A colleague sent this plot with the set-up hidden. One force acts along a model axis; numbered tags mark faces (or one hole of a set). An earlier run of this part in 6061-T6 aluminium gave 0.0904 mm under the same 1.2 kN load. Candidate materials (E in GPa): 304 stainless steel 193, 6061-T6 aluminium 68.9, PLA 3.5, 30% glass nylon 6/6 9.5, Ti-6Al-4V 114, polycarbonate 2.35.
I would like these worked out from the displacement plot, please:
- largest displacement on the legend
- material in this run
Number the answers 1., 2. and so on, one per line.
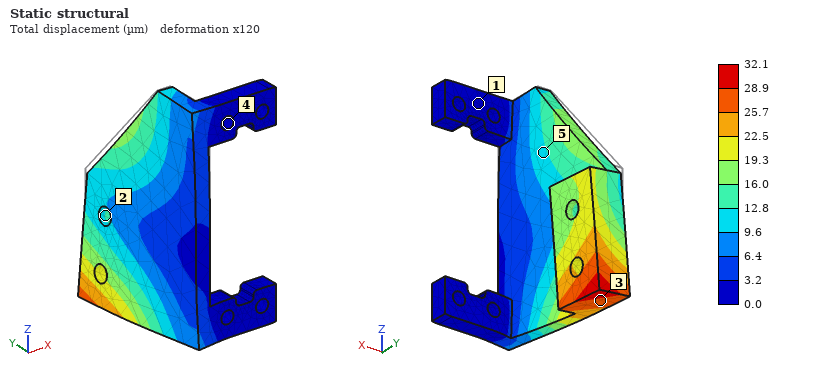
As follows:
1. 32.1 µm
2. 304 stainless steel
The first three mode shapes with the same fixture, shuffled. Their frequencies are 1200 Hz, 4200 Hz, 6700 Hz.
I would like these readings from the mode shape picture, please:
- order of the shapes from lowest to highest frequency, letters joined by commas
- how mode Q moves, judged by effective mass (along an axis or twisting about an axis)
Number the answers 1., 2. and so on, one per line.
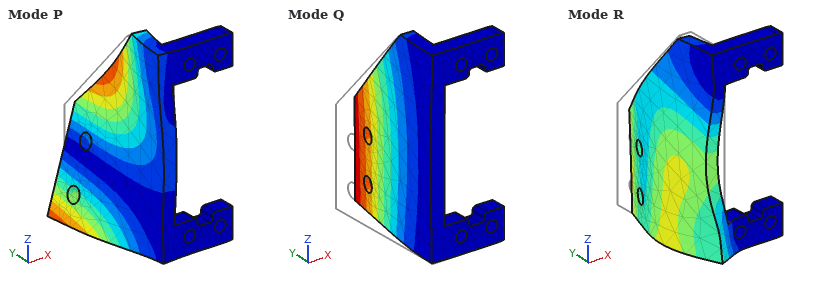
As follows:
1. Q, P, R
2. along X
